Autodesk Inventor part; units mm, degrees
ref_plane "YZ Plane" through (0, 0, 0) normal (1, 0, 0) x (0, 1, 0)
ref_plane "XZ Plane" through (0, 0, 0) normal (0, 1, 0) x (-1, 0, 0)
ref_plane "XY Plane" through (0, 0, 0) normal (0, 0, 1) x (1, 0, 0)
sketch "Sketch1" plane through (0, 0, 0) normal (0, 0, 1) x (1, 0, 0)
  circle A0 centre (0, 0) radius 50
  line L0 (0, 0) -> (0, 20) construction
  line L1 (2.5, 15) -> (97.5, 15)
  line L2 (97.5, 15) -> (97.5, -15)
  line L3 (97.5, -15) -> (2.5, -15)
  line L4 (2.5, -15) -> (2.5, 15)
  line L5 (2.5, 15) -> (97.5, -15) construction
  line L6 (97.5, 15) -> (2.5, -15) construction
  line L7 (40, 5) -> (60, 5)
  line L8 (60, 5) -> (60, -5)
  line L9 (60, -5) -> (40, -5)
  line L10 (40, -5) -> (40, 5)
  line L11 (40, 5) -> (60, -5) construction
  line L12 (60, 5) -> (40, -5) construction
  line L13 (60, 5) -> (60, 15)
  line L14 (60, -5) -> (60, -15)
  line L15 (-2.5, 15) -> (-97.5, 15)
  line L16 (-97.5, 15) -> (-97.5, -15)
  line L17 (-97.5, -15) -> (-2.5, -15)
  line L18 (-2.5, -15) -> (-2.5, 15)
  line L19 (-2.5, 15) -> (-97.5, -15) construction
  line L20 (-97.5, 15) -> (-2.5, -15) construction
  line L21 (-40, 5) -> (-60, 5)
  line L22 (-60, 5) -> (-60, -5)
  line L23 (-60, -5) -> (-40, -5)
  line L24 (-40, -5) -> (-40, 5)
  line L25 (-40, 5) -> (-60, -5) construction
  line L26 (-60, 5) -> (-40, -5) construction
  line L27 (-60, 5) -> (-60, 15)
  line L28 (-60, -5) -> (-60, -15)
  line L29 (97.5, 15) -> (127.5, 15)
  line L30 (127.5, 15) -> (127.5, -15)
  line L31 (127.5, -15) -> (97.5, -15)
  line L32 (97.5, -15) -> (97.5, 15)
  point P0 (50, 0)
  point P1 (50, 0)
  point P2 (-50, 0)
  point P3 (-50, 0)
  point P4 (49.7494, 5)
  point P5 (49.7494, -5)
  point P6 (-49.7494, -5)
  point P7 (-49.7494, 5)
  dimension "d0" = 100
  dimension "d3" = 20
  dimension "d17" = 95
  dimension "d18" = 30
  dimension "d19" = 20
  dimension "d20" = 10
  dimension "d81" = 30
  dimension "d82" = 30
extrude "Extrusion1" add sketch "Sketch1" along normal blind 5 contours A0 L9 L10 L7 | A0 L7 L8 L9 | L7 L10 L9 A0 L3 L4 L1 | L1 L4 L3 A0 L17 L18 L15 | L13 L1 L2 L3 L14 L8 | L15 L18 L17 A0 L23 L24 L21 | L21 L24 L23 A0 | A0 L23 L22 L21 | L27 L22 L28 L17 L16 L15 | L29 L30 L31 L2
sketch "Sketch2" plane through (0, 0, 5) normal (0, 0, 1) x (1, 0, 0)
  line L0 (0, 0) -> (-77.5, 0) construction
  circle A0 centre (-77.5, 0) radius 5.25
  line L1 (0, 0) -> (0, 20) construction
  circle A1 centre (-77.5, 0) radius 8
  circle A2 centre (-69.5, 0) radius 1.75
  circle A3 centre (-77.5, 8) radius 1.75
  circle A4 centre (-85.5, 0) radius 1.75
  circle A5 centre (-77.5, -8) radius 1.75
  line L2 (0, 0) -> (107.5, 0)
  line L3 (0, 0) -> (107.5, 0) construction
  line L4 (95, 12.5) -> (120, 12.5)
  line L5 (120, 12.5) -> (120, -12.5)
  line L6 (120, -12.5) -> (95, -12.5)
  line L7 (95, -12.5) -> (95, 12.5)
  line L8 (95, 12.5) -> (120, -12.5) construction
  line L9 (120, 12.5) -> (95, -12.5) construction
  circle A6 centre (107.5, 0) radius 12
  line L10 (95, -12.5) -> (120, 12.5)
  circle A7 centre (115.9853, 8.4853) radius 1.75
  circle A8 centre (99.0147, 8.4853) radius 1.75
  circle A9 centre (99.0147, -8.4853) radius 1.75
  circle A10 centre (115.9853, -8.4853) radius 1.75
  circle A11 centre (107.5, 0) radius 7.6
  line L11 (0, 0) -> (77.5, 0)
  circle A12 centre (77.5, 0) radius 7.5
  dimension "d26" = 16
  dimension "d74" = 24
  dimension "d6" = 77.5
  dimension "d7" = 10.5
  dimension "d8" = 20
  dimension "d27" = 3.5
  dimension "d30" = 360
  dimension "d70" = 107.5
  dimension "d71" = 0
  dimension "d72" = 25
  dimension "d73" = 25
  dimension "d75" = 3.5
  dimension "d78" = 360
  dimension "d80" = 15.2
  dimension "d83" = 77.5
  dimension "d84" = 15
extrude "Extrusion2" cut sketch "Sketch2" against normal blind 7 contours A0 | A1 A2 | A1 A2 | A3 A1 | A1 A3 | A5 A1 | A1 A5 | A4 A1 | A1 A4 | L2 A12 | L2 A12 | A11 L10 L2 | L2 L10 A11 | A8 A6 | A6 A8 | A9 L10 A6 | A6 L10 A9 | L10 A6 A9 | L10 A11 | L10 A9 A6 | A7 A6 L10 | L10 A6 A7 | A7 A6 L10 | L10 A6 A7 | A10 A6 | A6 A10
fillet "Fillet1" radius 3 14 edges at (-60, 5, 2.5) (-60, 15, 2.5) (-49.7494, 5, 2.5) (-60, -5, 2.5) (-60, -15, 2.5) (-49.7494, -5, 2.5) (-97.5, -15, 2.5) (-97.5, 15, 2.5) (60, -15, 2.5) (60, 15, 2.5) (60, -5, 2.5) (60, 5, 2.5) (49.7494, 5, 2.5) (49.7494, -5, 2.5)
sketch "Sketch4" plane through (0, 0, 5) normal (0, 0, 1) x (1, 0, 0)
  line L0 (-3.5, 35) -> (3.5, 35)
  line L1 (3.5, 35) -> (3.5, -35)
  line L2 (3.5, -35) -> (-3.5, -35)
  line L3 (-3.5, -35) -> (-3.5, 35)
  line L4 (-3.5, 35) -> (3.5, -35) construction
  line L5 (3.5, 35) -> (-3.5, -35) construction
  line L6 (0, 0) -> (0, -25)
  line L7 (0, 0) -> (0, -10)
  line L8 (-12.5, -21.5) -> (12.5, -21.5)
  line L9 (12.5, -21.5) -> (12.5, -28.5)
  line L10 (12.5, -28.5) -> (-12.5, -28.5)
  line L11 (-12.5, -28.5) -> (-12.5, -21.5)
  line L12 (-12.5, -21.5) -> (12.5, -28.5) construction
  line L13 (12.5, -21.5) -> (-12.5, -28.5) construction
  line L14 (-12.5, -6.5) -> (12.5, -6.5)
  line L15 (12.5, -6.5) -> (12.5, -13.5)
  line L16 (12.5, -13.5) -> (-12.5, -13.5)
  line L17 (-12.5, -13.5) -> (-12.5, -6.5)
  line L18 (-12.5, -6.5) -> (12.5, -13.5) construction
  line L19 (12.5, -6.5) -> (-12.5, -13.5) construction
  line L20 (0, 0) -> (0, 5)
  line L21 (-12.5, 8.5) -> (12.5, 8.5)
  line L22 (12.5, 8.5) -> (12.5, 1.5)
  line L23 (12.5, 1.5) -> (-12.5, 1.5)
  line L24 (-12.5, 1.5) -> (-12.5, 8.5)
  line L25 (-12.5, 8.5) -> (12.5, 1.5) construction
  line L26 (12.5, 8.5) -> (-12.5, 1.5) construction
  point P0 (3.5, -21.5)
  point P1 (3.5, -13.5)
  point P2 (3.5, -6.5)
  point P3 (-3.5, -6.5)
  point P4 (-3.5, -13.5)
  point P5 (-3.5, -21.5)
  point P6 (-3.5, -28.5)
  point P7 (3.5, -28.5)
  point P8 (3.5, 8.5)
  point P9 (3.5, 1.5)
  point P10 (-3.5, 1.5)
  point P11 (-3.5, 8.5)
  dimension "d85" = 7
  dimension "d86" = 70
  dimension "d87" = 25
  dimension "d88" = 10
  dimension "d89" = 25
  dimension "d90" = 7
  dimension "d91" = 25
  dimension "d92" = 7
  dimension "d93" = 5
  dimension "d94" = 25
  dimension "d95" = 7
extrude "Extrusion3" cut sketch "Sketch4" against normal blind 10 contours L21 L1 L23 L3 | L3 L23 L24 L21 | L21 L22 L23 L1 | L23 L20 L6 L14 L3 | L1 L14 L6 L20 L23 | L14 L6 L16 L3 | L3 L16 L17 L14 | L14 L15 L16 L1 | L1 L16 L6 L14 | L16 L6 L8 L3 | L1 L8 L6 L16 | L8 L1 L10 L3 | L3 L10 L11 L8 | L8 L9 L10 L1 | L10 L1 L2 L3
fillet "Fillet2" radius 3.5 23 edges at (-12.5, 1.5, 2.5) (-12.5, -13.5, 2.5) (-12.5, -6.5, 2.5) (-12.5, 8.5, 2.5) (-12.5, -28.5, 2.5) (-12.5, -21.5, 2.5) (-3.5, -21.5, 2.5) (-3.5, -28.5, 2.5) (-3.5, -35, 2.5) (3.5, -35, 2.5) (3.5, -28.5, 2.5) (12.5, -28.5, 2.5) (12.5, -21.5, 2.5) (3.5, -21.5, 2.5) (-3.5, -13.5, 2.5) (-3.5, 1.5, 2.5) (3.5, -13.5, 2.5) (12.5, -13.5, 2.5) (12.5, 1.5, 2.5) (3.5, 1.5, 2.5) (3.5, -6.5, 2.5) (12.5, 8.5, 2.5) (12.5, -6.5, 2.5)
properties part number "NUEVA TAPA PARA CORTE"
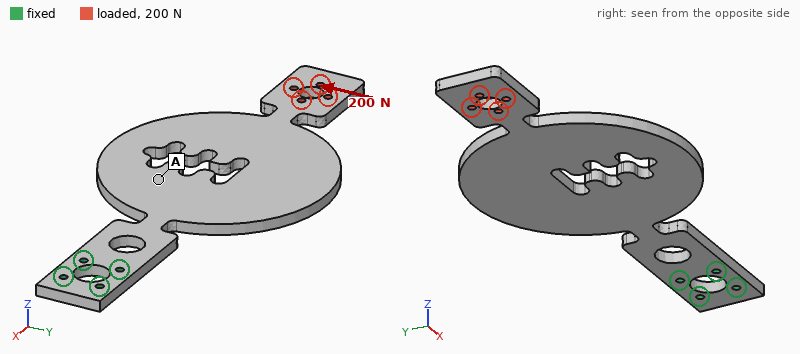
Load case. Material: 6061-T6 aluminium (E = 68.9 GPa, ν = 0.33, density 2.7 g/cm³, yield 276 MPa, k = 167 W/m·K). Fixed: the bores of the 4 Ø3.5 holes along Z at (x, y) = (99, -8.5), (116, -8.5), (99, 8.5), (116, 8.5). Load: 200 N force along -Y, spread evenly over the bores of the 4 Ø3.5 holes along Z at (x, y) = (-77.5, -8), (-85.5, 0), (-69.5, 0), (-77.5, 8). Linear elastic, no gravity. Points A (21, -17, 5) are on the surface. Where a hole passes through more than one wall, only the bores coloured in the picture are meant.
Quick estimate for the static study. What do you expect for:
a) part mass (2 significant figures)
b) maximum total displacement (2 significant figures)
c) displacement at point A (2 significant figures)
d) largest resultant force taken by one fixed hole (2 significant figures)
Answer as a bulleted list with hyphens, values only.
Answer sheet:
- 140 g
- 2.5 mm
- 0.62 mm
- 1.6 kN
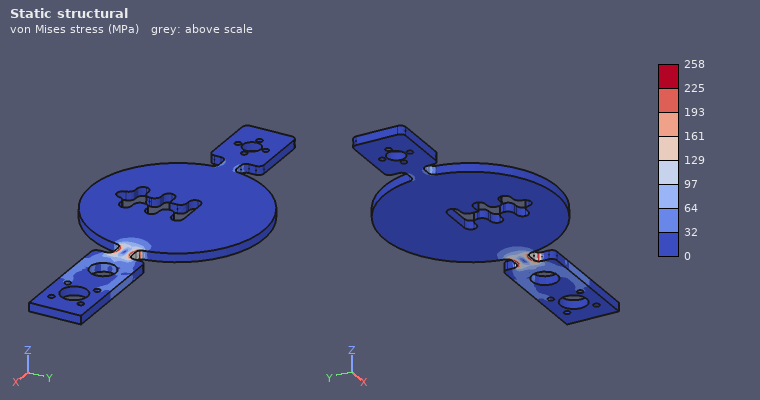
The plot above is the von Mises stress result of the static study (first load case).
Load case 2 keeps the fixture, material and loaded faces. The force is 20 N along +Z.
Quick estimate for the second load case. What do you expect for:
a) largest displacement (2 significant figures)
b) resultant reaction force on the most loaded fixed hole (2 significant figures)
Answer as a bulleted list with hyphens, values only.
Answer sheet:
- 2.8 mm
- 21 N
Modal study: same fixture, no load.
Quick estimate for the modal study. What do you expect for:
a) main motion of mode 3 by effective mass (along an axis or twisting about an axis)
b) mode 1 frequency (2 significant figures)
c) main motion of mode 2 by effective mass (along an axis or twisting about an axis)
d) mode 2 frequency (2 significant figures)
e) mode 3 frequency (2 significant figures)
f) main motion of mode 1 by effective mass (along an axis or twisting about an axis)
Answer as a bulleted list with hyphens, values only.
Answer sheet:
- twisting about X
- 76 Hz
- along Y
- 250 Hz
- 310 Hz
- along Z
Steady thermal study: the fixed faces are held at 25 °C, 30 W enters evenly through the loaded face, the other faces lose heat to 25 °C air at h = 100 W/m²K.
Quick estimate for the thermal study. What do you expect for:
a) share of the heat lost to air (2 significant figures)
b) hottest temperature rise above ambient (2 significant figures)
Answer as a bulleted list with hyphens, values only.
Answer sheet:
- 98 %
- 61 K
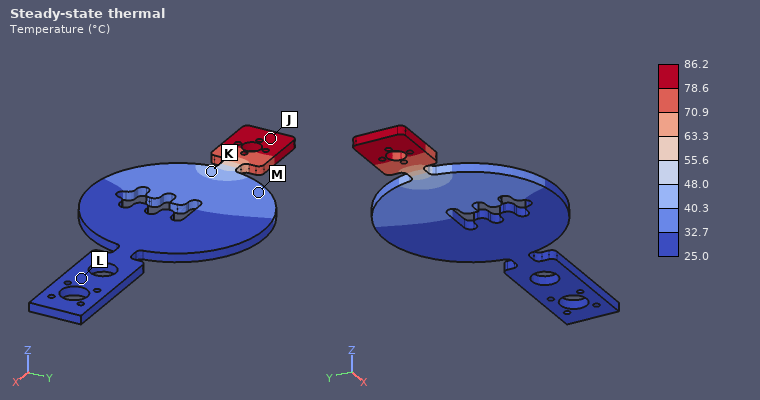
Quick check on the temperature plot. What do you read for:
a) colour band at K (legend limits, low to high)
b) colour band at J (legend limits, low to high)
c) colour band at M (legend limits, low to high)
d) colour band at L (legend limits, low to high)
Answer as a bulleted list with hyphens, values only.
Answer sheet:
- 40.3 to 48.0 °C
- 78.6 to 86.2 °C
- 32.7 to 40.3 °C
- 25.0 to 32.7 °C
